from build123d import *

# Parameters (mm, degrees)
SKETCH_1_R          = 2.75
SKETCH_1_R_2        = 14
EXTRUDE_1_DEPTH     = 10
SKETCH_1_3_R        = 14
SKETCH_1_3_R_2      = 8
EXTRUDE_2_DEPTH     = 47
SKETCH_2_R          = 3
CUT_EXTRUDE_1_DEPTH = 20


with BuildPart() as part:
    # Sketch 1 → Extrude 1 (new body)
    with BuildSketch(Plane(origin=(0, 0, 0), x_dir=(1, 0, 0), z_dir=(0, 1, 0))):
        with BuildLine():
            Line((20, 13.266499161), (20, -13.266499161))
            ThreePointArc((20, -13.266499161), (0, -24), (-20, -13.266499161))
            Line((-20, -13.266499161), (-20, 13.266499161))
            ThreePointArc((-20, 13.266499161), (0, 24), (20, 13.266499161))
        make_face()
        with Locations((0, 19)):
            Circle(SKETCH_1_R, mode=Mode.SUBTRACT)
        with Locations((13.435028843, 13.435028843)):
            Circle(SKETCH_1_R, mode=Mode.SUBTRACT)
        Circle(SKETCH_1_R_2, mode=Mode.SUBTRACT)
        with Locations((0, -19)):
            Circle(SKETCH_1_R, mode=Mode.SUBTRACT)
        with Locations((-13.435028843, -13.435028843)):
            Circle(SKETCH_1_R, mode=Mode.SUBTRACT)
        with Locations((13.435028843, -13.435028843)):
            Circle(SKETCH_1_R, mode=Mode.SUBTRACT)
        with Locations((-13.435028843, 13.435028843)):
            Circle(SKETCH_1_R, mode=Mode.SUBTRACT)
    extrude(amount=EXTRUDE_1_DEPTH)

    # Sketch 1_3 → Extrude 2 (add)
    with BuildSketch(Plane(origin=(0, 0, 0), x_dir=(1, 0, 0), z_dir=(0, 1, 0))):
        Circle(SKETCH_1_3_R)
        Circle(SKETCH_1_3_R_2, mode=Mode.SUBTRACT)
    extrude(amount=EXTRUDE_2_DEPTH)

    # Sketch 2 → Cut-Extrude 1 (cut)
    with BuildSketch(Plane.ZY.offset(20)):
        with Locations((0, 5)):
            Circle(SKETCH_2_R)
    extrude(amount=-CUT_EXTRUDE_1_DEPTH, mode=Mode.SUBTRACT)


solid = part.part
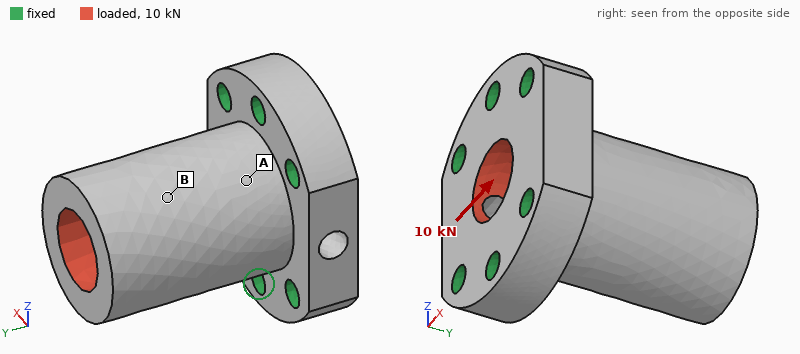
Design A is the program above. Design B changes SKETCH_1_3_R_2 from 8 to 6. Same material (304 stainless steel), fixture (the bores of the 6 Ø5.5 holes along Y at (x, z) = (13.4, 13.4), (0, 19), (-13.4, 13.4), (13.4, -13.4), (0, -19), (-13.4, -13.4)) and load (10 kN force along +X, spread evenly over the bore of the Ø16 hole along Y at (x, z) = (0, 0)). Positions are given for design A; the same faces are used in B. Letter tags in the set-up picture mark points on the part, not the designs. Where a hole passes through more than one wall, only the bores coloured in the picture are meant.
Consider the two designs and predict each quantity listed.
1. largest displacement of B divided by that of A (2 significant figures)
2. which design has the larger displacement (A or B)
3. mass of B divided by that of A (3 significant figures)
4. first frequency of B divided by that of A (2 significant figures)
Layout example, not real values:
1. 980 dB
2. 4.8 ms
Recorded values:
1. 0.90
2. A
3. 1.14
4. 0.97
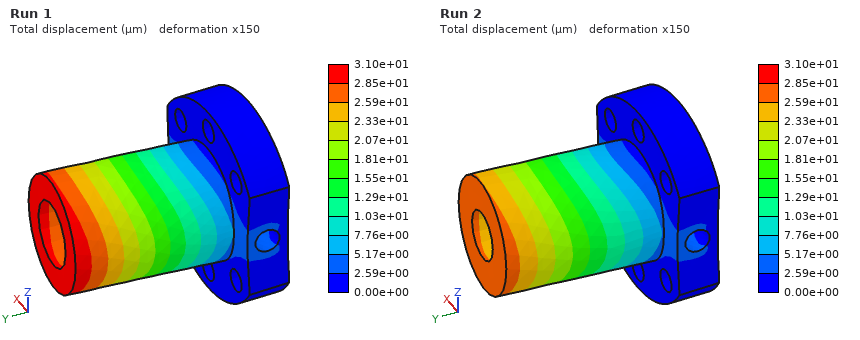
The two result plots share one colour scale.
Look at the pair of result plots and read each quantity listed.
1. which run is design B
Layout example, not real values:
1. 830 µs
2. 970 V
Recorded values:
1. Run 2
